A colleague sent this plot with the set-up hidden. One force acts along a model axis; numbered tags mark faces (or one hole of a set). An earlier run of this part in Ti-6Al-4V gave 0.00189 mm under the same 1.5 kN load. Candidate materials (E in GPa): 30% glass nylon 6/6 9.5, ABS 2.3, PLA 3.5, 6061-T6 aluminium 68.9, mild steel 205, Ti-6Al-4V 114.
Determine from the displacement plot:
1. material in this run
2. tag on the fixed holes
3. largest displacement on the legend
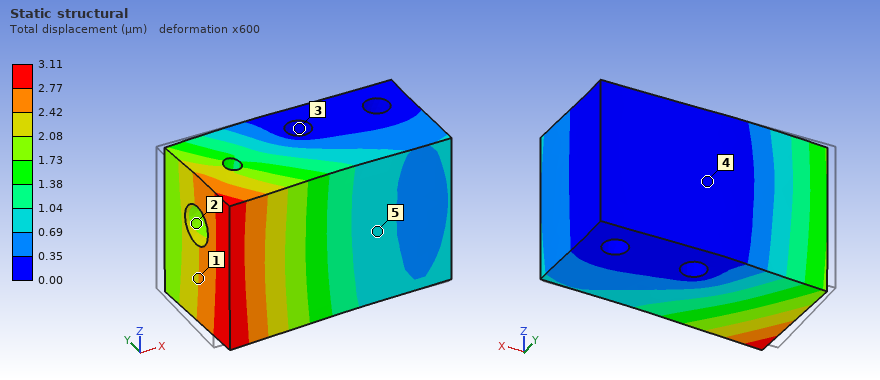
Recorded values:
6061-T6 aluminium
3
3.11 µm
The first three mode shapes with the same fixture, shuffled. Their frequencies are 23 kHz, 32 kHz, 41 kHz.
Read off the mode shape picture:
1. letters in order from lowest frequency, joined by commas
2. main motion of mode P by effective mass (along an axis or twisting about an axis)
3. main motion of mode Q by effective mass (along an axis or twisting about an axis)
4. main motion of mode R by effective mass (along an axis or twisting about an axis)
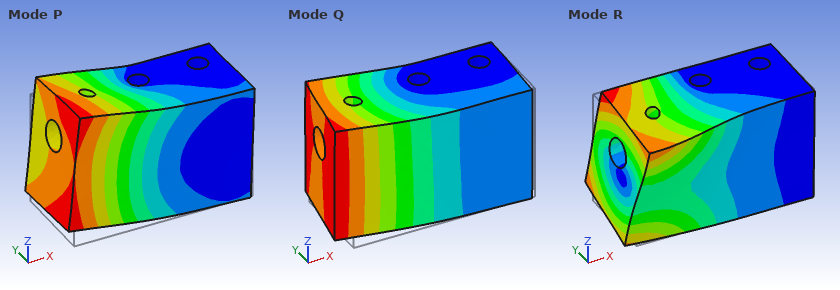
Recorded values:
Q, P, R
along Z
along Y
twisting about X
